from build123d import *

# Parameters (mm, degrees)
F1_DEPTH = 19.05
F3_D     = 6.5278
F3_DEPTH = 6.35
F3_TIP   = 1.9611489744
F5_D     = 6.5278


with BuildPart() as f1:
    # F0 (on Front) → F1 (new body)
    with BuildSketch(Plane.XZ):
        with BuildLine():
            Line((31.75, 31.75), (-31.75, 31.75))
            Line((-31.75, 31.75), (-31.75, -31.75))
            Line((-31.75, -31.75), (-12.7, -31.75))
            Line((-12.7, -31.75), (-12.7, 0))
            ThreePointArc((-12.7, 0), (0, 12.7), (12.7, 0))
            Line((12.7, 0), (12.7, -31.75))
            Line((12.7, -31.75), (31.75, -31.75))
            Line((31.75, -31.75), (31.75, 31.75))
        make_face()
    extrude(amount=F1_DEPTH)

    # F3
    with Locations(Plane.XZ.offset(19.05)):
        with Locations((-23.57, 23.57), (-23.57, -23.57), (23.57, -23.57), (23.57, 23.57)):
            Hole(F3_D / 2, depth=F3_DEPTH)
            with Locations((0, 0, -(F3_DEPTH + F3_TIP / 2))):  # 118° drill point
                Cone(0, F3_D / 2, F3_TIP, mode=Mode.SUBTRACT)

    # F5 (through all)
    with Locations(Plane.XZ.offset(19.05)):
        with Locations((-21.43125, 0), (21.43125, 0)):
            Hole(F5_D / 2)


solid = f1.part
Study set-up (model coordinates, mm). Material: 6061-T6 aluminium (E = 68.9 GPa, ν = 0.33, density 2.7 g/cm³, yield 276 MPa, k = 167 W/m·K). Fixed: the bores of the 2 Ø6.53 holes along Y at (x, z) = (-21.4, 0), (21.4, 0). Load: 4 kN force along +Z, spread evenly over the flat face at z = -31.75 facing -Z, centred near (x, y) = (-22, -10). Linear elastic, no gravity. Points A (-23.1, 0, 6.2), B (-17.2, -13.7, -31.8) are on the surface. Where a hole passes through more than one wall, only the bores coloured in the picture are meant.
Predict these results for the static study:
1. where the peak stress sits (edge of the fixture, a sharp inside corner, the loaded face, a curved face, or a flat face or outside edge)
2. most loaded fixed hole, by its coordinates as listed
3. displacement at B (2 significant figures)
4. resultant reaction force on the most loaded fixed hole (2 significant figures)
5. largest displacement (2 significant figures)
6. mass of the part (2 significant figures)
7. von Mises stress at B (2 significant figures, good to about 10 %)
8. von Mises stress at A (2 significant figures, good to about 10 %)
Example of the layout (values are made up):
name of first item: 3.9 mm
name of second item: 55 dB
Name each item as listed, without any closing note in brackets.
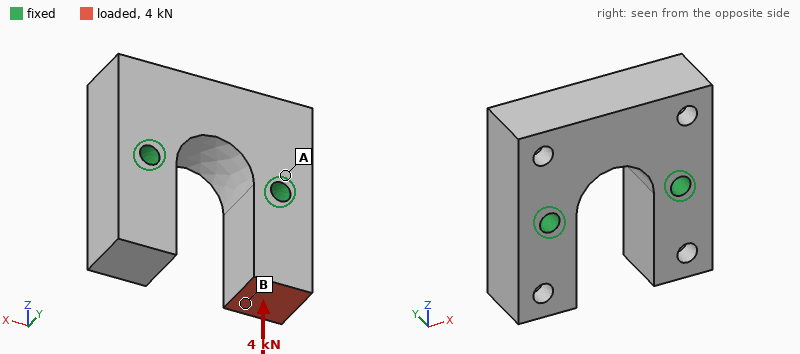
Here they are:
where the peak stress sits: a curved face
most loaded fixed hole, by its coordinates as listed: (-21.4, 0)
displacement at B: 5.6 µm
resultant reaction force on the most loaded fixed hole: 4.0 kN
largest displacement: 7.2 µm
mass of the part: 150 g
von Mises stress at B: 12 MPa
von Mises stress at A: 3.6 MPa
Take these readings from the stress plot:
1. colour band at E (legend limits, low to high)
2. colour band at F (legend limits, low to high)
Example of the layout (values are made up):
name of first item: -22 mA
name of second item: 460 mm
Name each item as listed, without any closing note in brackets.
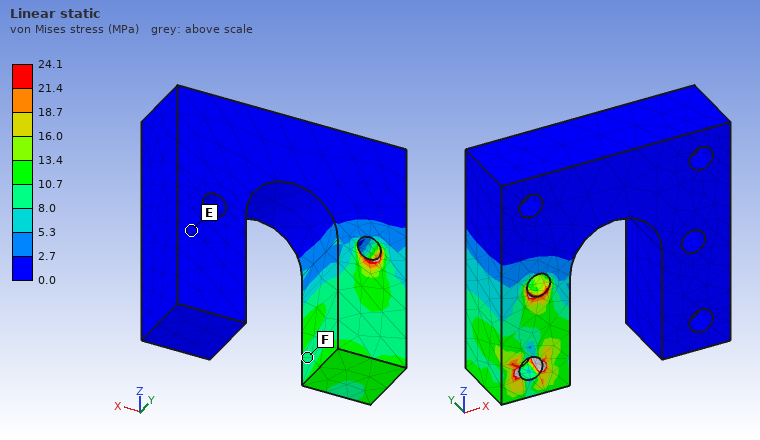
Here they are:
colour band at E: 0.0 to 2.7 MPa
colour band at F: 8.0 to 10.7 MPa
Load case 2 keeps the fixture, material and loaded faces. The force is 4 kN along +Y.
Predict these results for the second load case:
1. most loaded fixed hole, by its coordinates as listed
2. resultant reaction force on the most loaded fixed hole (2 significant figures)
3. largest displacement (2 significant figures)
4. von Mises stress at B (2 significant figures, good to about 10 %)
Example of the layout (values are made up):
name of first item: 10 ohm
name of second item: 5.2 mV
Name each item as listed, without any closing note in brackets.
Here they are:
most loaded fixed hole, by its coordinates as listed: (-21.4, 0)
resultant reaction force on the most loaded fixed hole: 4.1 kN
largest displacement: 78 µm
von Mises stress at B: 25 MPa
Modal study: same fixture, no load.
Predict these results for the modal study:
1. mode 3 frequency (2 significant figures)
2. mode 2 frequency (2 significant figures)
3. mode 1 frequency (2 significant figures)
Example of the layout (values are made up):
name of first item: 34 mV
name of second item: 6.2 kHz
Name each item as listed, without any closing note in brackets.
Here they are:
mode 3 frequency: 11 kHz
mode 2 frequency: 10 kHz
mode 1 frequency: 10 kHz
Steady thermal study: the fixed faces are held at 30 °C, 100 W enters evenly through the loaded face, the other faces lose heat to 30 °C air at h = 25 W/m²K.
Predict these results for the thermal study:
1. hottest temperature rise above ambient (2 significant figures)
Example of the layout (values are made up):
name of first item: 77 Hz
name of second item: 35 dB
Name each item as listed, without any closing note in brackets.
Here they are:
hottest temperature rise above ambient: 54 K
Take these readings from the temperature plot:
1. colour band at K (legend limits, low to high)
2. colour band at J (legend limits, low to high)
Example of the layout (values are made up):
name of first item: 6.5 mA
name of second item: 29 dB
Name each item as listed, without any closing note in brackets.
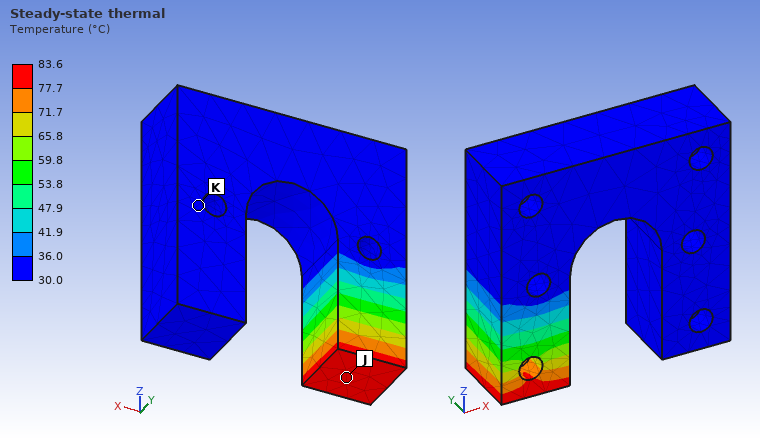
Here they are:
colour band at K: 30.0 to 36.0 °C
colour band at J: 77.7 to 83.6 °C
